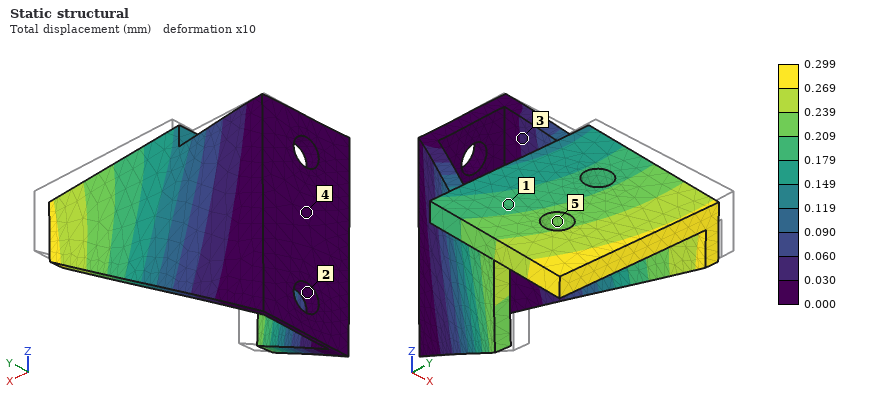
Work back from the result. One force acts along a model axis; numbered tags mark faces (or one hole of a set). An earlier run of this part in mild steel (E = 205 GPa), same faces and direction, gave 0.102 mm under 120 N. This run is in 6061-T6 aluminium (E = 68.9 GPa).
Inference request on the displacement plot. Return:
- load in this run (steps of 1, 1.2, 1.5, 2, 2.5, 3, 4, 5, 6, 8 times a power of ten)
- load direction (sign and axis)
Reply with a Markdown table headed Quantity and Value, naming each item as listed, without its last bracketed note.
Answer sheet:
| Quantity | Value |
|---|---|
| load in this run | 120 N |
| load direction | -Y |
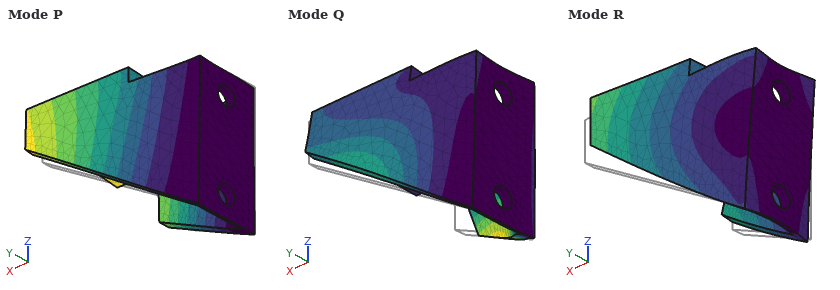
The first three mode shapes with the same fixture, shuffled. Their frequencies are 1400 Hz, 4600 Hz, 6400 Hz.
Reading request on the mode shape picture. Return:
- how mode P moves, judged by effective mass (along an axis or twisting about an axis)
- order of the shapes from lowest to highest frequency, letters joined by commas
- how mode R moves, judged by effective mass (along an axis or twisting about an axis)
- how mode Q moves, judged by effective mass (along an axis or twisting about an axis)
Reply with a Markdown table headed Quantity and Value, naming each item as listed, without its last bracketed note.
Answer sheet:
| Quantity | Value |
|---|---|
| how mode P moves, judged by effective mass | along Y |
| order of the shapes from lowest to highest frequency, letters joined by commas | P, R, Q |
| how mode R moves, judged by effective mass | along Z |
| how mode Q moves, judged by effective mass | along X |
